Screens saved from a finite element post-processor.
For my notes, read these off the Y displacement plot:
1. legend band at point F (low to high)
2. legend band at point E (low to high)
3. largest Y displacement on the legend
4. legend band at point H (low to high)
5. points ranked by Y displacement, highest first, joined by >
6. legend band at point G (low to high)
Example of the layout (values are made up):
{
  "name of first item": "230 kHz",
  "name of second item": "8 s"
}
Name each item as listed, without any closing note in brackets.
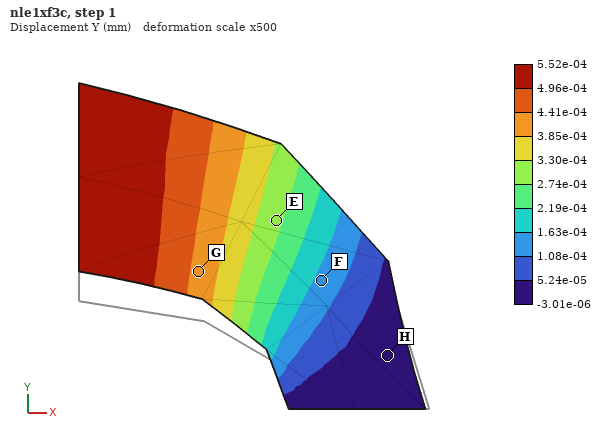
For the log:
{
  "legend band at point F": "1.08e-04 to 1.63e-04 mm",
  "legend band at point E": "2.74e-04 to 3.30e-04 mm",
  "largest Y displacement on the legend": "5.52e-04 mm",
  "legend band at point H": "-3.01e-06 to 5.24e-05 mm",
  "points ranked by Y displacement, highest first, joined by >": "G > E > F > H",
  "legend band at point G": "3.85e-04 to 4.41e-04 mm"
}
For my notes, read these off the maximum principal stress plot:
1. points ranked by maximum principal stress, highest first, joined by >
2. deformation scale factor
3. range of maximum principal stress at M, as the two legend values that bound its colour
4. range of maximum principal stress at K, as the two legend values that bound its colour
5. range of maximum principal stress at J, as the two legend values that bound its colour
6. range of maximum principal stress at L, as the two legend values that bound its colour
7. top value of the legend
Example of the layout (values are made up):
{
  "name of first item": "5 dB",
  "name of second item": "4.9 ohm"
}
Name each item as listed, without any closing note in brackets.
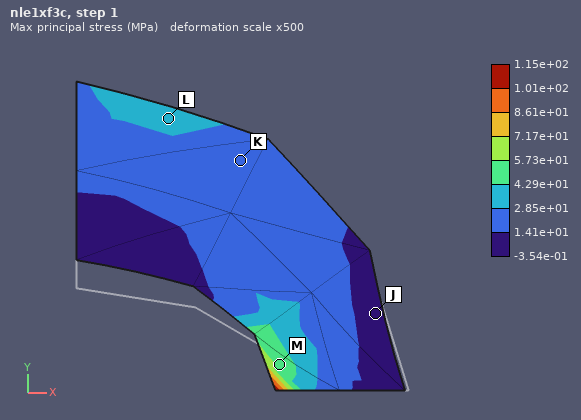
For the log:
{
  "points ranked by maximum principal stress, highest first, joined by >": "M > L > K > J",
  "deformation scale factor": "500",
  "range of maximum principal stress at M, as the two legend values that bound its colour": "4.29e+01 to 5.73e+01 MPa",
  "range of maximum principal stress at K, as the two legend values that bound its colour": "1.41e+01 to 2.85e+01 MPa",
  "range of maximum principal stress at J, as the two legend values that bound its colour": "-3.54e-01 to 1.41e+01 MPa",
  "range of maximum principal stress at L, as the two legend values that bound its colour": "2.85e+01 to 4.29e+01 MPa",
  "top value of the legend": "1.15e+02 MPa"
}
